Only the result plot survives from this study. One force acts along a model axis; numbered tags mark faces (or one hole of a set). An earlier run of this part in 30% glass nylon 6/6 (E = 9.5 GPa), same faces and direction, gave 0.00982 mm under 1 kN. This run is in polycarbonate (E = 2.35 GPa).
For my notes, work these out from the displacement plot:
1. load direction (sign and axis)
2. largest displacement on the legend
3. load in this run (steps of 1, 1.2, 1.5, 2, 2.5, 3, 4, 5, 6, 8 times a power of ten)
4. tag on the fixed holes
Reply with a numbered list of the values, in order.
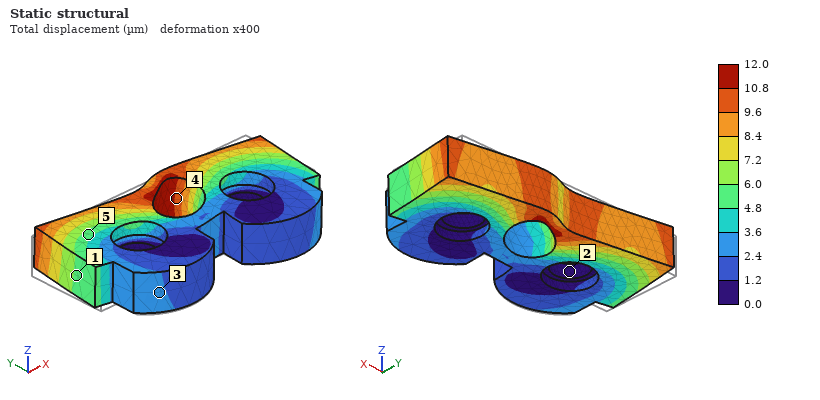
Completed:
1. +X
2. 12.0 µm
3. 300 N
4. 2
